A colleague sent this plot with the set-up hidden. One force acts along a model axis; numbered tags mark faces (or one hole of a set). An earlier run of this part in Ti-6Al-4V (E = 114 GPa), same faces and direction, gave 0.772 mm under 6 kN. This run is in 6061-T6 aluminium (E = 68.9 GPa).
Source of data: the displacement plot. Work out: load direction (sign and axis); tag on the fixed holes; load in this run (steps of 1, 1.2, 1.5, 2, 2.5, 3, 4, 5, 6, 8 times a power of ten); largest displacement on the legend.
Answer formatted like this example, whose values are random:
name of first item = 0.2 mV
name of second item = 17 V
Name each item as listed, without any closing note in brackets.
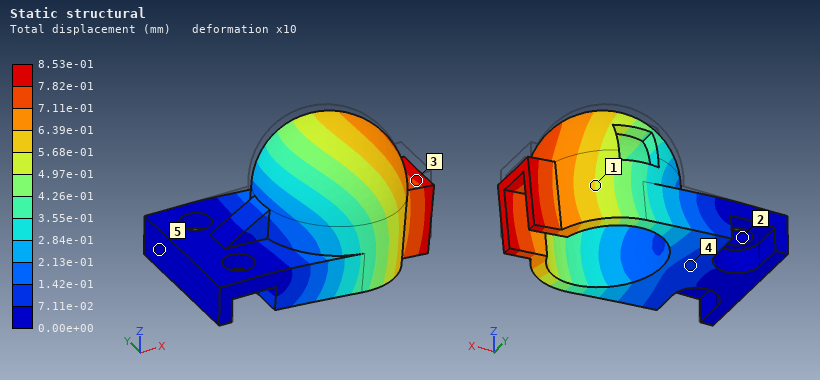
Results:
load direction = -Z
tag on the fixed holes = 2
load in this run = 4 kN
largest displacement on the legend = 8.53e-01 mm
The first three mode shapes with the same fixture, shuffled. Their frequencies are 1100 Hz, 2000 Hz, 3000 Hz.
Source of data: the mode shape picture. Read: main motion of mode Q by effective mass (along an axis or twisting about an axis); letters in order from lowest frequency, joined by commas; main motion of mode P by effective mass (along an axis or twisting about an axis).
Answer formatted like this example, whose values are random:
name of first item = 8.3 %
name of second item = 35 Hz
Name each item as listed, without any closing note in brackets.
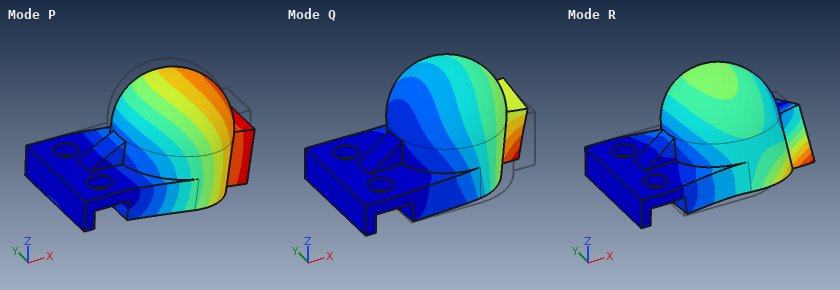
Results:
main motion of mode Q by effective mass = along Y
letters in order from lowest frequency, joined by commas = P, Q, R
main motion of mode P by effective mass = along Z
